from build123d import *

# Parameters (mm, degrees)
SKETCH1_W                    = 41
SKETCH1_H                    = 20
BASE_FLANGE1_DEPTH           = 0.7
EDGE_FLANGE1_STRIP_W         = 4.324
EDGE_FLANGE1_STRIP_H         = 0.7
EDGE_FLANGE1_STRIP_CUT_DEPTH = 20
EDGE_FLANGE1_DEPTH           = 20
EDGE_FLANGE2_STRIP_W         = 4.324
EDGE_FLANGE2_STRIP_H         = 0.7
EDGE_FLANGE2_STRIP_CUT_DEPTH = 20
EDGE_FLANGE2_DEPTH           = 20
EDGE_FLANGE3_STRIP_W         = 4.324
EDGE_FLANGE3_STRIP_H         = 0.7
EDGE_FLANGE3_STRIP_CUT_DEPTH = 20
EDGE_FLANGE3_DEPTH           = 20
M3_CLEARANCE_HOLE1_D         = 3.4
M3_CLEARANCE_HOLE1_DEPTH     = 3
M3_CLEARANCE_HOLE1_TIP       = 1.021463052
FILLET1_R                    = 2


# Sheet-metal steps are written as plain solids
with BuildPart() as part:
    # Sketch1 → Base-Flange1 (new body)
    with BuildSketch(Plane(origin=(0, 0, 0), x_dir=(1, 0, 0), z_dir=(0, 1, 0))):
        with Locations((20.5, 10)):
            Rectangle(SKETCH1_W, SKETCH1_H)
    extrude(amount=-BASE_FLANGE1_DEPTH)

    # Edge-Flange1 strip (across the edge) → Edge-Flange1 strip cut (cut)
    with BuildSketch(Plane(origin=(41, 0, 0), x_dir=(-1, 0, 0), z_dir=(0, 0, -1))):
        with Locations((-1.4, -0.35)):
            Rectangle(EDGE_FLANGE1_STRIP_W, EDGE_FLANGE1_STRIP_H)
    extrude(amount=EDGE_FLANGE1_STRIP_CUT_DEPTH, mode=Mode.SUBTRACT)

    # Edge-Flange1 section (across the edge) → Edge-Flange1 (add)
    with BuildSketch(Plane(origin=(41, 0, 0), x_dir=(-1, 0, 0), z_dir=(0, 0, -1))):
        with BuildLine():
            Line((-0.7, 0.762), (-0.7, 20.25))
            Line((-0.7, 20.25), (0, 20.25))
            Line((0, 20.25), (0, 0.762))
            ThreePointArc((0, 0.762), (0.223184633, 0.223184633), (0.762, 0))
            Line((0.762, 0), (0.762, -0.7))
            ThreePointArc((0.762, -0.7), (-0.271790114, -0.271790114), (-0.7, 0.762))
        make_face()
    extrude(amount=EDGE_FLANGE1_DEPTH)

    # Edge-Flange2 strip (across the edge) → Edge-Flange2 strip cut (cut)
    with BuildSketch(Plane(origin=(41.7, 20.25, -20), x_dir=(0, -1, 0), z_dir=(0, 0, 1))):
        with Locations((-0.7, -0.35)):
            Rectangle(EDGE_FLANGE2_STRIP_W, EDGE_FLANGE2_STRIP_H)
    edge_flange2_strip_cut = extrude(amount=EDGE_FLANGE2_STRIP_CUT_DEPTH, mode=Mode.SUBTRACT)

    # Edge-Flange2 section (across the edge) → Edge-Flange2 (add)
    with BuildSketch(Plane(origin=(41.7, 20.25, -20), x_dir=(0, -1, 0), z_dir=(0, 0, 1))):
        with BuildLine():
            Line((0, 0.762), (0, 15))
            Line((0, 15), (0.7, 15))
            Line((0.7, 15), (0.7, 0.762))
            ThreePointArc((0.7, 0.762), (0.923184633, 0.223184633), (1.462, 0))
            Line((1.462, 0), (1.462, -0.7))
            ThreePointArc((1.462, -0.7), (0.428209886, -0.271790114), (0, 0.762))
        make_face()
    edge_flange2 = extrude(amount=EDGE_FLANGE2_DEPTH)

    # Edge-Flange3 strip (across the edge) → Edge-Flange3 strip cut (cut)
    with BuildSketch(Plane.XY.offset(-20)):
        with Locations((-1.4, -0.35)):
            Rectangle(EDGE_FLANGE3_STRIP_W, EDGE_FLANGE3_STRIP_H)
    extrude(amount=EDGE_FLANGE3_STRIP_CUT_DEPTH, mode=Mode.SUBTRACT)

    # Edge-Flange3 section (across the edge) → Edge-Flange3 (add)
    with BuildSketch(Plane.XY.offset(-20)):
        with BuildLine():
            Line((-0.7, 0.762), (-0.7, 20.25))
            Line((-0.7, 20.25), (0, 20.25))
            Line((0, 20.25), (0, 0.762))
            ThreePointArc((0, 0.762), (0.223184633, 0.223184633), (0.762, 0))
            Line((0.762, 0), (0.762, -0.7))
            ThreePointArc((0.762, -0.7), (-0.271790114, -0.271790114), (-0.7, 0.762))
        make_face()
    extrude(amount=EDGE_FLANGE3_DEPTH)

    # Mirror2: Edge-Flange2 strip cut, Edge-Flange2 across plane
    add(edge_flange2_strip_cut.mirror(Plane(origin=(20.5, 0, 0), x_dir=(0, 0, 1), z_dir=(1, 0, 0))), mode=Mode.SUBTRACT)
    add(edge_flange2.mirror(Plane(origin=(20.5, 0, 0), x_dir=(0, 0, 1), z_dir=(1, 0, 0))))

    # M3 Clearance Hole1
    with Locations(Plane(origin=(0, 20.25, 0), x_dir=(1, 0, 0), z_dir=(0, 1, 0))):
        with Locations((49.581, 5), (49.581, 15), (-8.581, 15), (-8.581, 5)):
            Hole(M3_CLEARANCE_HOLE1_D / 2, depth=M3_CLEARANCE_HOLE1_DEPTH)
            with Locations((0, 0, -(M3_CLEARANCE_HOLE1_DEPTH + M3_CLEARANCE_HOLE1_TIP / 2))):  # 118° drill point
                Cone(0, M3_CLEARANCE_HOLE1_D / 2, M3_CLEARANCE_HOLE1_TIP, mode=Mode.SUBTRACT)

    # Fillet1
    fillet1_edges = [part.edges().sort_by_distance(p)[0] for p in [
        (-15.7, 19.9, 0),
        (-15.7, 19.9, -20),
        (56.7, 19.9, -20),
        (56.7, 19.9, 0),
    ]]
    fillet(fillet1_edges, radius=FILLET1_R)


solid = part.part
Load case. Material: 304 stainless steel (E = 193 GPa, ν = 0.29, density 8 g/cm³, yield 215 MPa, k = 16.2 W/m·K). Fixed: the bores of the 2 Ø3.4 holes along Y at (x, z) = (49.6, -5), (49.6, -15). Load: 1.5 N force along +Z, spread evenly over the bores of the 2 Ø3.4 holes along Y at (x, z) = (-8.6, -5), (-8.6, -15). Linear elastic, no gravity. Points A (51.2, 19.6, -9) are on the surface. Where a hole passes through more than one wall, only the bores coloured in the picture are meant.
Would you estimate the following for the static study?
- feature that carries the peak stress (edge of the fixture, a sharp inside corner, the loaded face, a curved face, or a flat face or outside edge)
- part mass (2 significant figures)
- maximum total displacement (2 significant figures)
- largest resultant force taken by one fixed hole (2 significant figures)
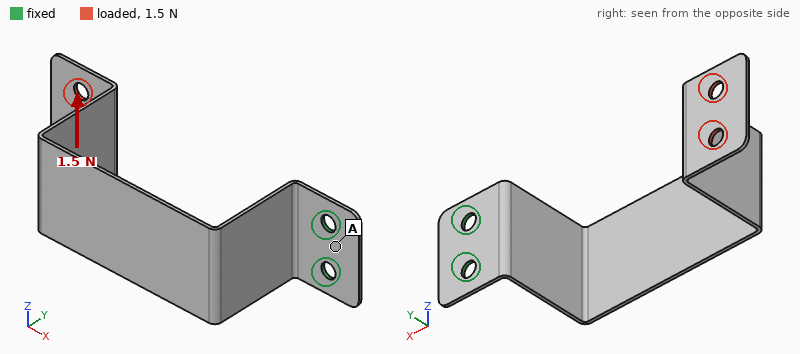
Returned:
a curved face
12 g
0.59 mm
7.1 N
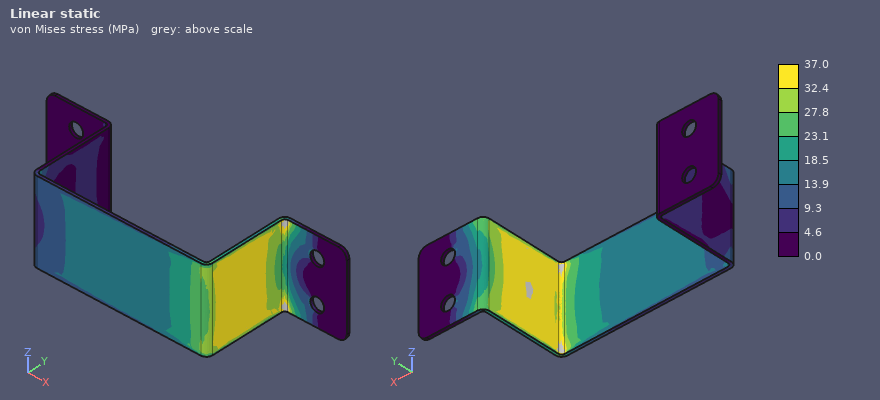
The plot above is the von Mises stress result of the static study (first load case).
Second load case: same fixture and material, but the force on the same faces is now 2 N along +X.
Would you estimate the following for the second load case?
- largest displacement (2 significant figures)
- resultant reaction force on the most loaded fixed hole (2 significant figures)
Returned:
0.87 mm
1.0 N
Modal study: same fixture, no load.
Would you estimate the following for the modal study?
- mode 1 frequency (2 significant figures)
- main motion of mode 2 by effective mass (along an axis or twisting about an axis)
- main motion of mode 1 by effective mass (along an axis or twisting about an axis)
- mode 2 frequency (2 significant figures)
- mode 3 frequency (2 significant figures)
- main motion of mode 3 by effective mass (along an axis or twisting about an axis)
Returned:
79 Hz
along Z
along Y
150 Hz
260 Hz
along X
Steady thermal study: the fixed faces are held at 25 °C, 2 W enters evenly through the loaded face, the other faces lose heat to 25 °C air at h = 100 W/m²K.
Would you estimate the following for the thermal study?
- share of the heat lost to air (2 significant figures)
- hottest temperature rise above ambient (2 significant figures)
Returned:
100 %
42 K
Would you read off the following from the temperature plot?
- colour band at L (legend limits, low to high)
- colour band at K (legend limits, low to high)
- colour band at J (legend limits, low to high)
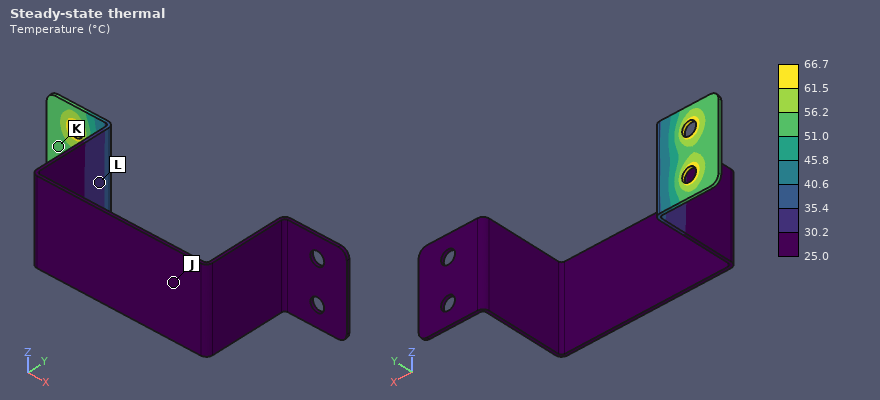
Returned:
30.2 to 35.4 °C
51.0 to 56.2 °C
25.0 to 30.2 °C
